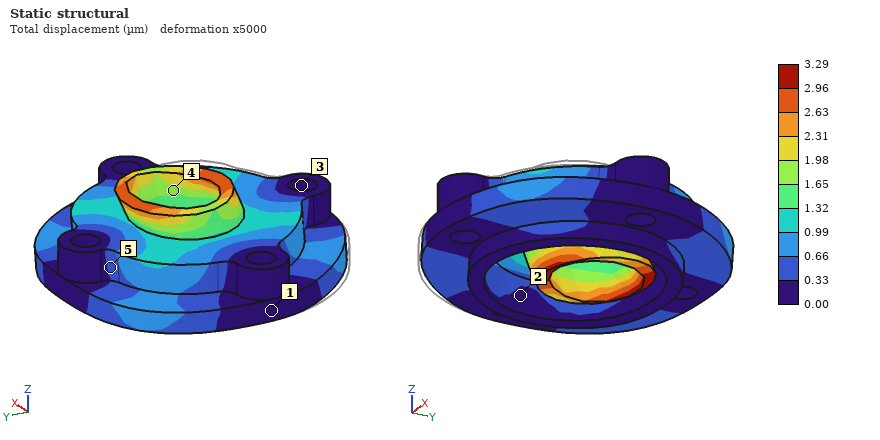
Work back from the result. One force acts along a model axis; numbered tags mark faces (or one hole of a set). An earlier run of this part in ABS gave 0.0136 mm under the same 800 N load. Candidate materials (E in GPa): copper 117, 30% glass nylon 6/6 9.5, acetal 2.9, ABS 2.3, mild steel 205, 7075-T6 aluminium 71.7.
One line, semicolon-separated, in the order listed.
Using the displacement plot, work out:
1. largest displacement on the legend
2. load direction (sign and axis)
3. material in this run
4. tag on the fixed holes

3.29 µm; +Y; 30% glass nylon 6/6; 3
